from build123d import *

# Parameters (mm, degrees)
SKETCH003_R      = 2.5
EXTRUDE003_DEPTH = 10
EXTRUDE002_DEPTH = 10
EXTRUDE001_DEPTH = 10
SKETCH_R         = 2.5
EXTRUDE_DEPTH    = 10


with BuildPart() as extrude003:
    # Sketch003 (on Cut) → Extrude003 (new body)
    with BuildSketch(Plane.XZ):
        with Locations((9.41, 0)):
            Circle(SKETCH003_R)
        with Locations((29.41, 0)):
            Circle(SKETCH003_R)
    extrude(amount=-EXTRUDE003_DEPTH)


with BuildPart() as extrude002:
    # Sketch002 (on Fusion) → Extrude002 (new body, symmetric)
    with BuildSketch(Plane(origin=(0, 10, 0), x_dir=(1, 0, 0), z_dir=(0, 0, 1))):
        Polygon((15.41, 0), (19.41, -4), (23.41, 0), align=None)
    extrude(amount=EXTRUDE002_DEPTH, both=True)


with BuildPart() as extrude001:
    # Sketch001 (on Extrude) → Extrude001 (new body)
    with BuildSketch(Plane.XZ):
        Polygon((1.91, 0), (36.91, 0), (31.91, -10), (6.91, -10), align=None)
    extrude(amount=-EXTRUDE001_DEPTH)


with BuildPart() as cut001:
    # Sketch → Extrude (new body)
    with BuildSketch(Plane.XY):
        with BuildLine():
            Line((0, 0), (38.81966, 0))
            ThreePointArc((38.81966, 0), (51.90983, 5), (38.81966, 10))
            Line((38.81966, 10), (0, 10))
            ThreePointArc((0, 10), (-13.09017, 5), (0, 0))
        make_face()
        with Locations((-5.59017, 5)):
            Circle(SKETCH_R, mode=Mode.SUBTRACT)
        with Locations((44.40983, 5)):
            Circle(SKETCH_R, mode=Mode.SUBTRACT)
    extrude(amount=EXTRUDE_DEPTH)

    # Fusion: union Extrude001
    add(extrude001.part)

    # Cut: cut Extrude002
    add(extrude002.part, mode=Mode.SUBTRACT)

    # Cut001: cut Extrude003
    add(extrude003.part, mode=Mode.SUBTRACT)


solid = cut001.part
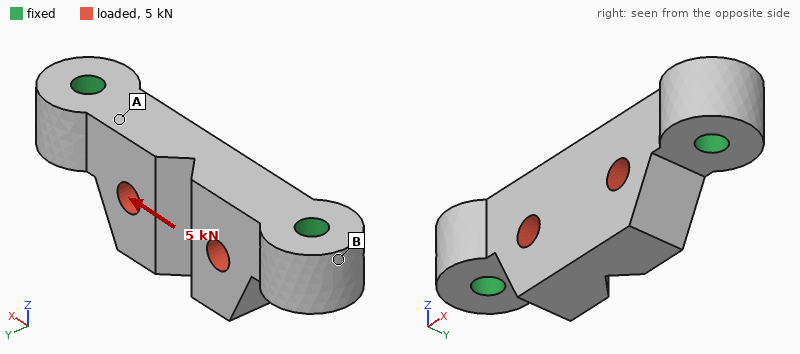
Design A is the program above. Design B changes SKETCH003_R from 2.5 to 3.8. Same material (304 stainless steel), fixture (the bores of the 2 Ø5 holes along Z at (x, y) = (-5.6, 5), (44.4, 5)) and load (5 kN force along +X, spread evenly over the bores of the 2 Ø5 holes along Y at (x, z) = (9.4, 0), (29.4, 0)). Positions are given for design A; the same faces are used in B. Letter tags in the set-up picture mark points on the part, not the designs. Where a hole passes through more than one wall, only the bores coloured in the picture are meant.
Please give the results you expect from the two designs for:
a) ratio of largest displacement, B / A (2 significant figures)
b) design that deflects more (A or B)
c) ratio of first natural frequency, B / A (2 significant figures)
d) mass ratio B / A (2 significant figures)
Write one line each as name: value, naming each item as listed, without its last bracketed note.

ratio of largest displacement, B / A: 1.4
design that deflects more: B
ratio of first natural frequency, B / A: 0.99
mass ratio B / A: 0.94
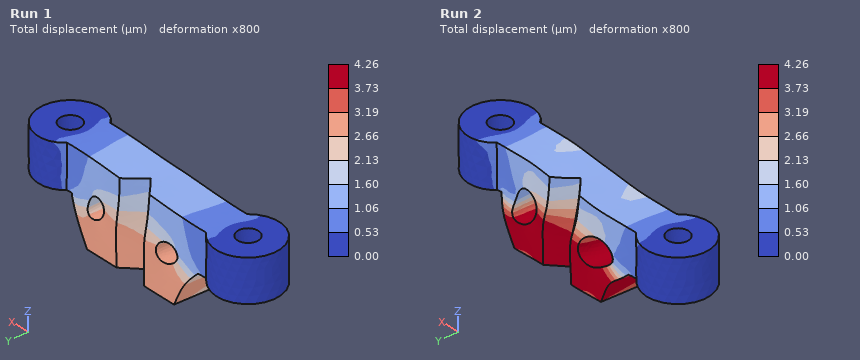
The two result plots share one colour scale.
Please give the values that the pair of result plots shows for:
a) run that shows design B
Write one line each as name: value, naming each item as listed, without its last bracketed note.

run that shows design B: Run 2
